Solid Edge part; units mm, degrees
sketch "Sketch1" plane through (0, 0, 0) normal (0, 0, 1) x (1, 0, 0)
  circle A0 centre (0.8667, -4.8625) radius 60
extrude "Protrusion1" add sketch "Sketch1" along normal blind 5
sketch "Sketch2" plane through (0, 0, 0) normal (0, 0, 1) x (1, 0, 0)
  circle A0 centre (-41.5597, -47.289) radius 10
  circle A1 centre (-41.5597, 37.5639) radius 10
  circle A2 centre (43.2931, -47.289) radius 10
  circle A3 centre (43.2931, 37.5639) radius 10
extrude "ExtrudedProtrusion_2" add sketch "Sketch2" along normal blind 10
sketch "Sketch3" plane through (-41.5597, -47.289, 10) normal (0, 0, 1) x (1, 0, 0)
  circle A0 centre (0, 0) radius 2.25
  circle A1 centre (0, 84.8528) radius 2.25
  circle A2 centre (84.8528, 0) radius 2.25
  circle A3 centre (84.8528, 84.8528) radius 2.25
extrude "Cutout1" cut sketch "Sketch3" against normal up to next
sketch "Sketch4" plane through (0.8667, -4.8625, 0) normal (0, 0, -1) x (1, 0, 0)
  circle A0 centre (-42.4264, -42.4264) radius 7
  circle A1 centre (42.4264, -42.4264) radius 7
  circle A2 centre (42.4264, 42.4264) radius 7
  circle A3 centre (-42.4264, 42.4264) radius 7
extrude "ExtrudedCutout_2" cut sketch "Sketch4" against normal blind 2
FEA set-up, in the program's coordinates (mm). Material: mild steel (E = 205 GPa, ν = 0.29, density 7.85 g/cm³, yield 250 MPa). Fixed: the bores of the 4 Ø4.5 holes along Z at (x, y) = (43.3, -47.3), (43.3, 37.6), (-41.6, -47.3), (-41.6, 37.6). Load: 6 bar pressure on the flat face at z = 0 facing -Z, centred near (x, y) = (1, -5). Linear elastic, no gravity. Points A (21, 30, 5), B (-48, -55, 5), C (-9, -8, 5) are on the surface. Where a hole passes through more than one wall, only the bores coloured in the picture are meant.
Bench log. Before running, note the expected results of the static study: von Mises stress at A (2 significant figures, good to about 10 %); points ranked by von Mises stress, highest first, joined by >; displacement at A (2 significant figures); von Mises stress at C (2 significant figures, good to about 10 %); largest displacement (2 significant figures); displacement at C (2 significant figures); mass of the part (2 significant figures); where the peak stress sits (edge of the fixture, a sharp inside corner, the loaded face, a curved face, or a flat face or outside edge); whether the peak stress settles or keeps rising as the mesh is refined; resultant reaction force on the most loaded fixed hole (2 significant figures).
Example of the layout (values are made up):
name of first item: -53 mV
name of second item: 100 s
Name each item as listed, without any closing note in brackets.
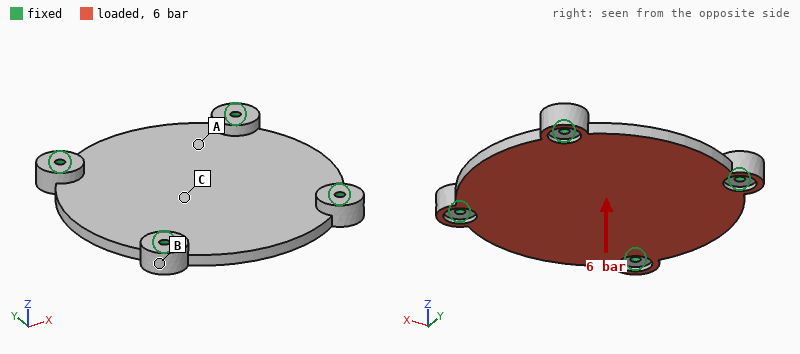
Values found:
von Mises stress at A: 22 MPa
points ranked by von Mises stress, highest first, joined by >: C > A > B
displacement at A: 29 µm
von Mises stress at C: 39 MPa
largest displacement: 72 µm
displacement at C: 70 µm
mass of the part: 510 g
where the peak stress sits: edge of the fixture
whether the peak stress settles or keeps rising as the mesh is refined: keeps rising
resultant reaction force on the most loaded fixed hole: 2.5 kN
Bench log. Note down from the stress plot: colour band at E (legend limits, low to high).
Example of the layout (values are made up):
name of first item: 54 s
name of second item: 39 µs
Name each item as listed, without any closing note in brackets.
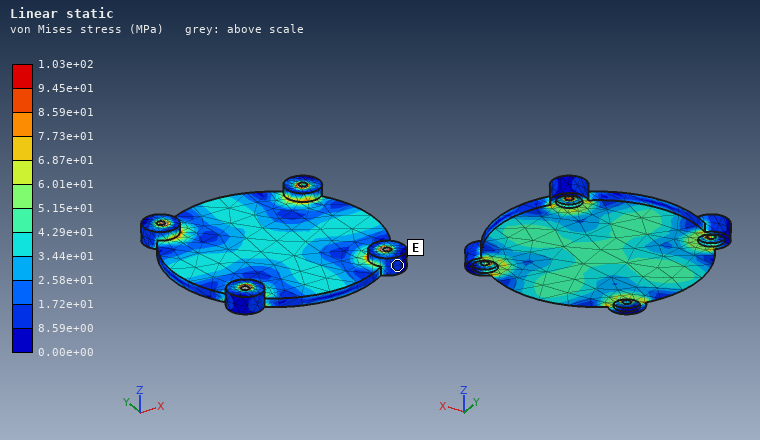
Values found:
colour band at E: 8.59e+00 to 1.72e+01 MPa
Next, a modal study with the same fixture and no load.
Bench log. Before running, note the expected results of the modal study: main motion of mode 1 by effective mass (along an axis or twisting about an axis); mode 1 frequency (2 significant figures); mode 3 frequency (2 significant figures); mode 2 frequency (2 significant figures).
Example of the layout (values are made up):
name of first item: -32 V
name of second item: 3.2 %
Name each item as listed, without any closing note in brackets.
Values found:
main motion of mode 1 by effective mass: along Z
mode 1 frequency: 2800 Hz
mode 3 frequency: 4100 Hz
mode 2 frequency: 4100 Hz
